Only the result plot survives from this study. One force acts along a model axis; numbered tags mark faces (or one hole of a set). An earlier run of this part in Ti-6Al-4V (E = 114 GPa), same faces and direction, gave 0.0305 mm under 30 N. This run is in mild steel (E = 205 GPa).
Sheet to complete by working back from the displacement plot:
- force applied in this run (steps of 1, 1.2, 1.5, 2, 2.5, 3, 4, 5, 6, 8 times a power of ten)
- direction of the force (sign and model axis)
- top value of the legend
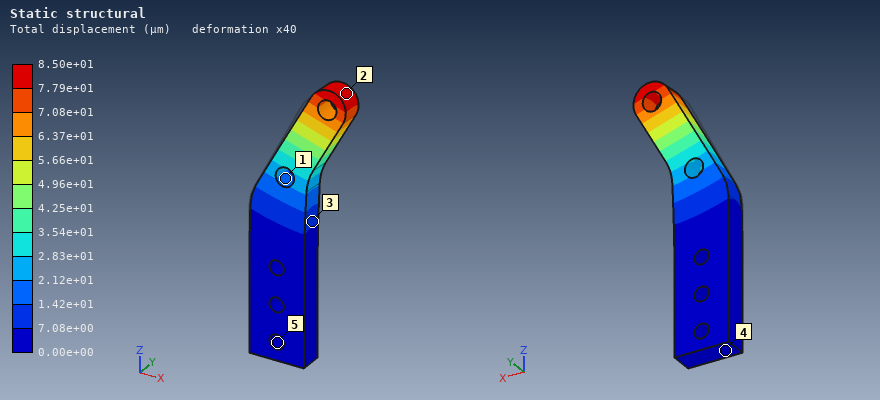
150 N
+Y
8.50e+01 µm
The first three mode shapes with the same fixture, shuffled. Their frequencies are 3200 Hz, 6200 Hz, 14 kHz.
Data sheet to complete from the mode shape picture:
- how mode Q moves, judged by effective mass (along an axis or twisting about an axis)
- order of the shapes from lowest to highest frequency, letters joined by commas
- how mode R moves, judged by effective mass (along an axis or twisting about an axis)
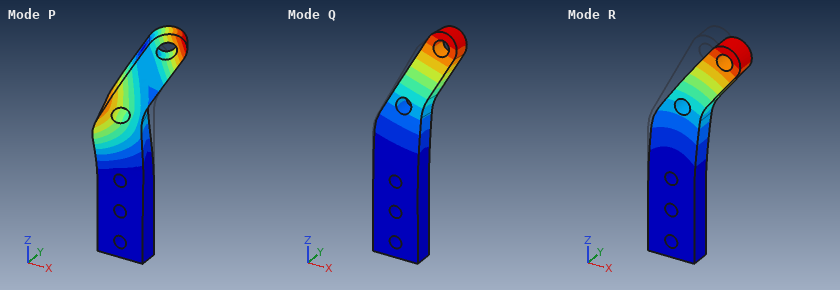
along Y
Q, R, P
along X
